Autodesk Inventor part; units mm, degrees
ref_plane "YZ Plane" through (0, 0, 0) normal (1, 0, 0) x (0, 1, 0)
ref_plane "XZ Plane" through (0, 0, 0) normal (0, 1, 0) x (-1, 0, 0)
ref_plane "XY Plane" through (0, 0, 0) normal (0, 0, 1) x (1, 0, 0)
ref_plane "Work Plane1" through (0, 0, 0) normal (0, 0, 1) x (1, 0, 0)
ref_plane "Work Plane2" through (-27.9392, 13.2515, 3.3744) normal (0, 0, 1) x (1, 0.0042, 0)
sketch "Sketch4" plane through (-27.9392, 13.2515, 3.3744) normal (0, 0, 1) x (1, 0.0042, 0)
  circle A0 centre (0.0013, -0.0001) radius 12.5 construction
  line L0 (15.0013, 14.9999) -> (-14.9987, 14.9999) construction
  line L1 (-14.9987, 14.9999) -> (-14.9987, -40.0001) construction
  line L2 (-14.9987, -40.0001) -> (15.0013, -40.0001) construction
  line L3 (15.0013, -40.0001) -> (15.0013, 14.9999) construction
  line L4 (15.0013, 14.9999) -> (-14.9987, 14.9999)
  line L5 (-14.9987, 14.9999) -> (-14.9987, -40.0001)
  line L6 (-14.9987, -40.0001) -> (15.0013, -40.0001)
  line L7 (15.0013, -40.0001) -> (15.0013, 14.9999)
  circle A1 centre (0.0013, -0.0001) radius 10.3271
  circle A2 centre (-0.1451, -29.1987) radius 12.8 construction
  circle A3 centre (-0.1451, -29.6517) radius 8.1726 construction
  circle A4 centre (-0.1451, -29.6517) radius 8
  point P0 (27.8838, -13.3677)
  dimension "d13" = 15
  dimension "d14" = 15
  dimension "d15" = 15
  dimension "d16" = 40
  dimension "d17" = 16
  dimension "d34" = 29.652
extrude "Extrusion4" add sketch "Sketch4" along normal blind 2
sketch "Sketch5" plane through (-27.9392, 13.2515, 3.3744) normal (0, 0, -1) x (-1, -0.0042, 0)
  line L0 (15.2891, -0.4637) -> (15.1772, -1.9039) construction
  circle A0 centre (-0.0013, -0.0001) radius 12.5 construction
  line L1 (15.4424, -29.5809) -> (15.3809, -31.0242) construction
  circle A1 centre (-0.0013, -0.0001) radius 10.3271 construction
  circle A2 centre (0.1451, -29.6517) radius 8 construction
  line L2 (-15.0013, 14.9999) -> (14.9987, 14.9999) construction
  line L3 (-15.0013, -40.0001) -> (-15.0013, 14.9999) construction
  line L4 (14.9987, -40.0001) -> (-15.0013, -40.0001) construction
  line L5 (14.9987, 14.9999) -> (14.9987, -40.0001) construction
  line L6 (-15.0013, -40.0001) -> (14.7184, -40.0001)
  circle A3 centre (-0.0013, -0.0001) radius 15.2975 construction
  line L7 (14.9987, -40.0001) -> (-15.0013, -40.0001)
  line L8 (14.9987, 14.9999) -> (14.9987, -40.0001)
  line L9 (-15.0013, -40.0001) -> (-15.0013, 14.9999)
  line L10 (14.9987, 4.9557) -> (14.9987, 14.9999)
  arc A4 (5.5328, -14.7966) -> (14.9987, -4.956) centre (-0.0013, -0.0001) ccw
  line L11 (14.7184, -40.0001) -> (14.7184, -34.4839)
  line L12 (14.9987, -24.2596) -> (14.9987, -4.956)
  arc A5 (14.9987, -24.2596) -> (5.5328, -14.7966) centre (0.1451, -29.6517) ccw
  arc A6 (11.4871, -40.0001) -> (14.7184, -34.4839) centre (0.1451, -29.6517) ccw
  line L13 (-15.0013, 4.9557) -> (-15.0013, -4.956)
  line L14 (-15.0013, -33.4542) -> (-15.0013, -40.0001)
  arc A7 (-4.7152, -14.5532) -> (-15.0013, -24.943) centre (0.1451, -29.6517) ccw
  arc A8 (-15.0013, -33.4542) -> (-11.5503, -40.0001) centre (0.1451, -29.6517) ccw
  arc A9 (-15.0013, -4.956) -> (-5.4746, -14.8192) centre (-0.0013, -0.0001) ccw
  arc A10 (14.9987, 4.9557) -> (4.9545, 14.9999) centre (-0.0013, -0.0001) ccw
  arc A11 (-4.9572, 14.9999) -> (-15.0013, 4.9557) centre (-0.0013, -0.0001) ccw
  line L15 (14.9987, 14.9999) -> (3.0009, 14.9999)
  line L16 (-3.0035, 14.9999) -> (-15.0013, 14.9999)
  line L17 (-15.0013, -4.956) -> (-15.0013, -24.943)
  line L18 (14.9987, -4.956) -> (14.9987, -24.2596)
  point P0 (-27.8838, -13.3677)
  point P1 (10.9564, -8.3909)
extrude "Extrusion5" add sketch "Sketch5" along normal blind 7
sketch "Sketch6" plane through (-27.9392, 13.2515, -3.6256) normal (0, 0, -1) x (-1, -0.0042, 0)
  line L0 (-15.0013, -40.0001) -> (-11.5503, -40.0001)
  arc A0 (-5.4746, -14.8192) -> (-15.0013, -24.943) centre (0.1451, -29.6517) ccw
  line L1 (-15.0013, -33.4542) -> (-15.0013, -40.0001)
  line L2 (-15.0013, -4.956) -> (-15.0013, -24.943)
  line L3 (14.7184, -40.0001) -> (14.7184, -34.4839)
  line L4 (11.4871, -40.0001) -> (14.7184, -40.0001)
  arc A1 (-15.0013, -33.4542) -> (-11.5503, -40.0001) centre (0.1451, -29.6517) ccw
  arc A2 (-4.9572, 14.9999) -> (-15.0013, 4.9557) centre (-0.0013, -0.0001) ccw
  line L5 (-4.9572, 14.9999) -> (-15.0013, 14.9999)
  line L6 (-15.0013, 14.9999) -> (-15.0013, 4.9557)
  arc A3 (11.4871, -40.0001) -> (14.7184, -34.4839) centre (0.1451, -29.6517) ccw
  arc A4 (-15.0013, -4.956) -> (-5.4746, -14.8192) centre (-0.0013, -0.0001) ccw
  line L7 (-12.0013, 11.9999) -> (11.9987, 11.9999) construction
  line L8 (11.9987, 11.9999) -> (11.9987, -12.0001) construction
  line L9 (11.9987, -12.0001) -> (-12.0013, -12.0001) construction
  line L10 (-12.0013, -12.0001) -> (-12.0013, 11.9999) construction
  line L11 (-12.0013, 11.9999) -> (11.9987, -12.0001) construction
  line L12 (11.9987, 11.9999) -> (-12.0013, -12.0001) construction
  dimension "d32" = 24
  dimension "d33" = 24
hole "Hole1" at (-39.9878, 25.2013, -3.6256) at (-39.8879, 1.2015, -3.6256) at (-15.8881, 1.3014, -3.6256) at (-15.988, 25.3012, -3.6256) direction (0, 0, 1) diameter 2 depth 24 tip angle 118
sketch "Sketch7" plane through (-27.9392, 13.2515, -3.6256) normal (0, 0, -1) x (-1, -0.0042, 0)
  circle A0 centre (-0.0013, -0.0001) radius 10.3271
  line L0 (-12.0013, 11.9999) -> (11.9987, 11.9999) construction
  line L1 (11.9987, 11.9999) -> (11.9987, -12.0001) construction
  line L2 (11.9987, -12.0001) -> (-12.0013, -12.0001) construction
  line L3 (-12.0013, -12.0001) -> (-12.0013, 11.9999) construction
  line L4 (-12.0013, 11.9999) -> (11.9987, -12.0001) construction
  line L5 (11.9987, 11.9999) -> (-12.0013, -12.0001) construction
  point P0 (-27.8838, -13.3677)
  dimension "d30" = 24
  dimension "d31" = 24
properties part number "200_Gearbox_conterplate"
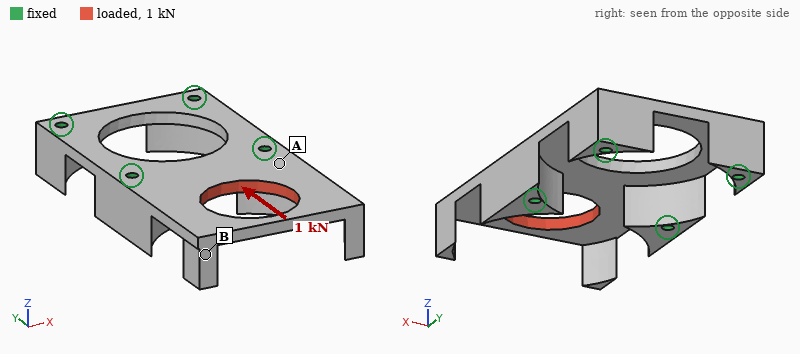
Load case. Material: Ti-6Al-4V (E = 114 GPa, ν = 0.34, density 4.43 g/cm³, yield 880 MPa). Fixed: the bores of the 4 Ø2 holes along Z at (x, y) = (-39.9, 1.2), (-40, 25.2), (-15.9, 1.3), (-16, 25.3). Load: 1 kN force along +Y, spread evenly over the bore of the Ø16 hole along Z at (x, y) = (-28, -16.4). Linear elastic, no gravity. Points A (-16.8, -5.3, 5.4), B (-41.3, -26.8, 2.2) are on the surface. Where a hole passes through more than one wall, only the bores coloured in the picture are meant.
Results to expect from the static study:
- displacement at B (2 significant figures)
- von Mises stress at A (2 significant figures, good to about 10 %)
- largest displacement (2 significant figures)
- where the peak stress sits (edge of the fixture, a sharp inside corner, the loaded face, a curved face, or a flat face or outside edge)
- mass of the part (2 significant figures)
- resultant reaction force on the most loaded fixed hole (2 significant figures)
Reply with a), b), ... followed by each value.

a) 10 µm
b) 28 MPa
c) 16 µm
d) a flat face or outside edge
e) 16 g
f) 500 N
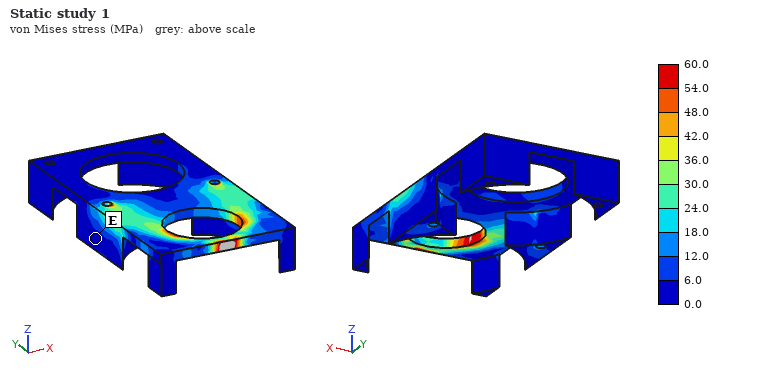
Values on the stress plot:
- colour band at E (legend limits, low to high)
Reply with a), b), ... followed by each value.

a) 0.0 to 6.0 MPa
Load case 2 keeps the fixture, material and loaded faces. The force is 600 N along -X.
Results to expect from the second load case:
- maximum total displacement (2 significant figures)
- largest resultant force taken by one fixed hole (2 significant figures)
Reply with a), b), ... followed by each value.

a) 29 µm
b) 480 N
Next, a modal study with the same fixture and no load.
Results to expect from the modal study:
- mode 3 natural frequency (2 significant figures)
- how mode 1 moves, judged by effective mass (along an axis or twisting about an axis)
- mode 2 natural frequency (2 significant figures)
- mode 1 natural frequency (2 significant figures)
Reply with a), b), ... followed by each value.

a) 9600 Hz
b) along Z
c) 4800 Hz
d) 2900 Hz
